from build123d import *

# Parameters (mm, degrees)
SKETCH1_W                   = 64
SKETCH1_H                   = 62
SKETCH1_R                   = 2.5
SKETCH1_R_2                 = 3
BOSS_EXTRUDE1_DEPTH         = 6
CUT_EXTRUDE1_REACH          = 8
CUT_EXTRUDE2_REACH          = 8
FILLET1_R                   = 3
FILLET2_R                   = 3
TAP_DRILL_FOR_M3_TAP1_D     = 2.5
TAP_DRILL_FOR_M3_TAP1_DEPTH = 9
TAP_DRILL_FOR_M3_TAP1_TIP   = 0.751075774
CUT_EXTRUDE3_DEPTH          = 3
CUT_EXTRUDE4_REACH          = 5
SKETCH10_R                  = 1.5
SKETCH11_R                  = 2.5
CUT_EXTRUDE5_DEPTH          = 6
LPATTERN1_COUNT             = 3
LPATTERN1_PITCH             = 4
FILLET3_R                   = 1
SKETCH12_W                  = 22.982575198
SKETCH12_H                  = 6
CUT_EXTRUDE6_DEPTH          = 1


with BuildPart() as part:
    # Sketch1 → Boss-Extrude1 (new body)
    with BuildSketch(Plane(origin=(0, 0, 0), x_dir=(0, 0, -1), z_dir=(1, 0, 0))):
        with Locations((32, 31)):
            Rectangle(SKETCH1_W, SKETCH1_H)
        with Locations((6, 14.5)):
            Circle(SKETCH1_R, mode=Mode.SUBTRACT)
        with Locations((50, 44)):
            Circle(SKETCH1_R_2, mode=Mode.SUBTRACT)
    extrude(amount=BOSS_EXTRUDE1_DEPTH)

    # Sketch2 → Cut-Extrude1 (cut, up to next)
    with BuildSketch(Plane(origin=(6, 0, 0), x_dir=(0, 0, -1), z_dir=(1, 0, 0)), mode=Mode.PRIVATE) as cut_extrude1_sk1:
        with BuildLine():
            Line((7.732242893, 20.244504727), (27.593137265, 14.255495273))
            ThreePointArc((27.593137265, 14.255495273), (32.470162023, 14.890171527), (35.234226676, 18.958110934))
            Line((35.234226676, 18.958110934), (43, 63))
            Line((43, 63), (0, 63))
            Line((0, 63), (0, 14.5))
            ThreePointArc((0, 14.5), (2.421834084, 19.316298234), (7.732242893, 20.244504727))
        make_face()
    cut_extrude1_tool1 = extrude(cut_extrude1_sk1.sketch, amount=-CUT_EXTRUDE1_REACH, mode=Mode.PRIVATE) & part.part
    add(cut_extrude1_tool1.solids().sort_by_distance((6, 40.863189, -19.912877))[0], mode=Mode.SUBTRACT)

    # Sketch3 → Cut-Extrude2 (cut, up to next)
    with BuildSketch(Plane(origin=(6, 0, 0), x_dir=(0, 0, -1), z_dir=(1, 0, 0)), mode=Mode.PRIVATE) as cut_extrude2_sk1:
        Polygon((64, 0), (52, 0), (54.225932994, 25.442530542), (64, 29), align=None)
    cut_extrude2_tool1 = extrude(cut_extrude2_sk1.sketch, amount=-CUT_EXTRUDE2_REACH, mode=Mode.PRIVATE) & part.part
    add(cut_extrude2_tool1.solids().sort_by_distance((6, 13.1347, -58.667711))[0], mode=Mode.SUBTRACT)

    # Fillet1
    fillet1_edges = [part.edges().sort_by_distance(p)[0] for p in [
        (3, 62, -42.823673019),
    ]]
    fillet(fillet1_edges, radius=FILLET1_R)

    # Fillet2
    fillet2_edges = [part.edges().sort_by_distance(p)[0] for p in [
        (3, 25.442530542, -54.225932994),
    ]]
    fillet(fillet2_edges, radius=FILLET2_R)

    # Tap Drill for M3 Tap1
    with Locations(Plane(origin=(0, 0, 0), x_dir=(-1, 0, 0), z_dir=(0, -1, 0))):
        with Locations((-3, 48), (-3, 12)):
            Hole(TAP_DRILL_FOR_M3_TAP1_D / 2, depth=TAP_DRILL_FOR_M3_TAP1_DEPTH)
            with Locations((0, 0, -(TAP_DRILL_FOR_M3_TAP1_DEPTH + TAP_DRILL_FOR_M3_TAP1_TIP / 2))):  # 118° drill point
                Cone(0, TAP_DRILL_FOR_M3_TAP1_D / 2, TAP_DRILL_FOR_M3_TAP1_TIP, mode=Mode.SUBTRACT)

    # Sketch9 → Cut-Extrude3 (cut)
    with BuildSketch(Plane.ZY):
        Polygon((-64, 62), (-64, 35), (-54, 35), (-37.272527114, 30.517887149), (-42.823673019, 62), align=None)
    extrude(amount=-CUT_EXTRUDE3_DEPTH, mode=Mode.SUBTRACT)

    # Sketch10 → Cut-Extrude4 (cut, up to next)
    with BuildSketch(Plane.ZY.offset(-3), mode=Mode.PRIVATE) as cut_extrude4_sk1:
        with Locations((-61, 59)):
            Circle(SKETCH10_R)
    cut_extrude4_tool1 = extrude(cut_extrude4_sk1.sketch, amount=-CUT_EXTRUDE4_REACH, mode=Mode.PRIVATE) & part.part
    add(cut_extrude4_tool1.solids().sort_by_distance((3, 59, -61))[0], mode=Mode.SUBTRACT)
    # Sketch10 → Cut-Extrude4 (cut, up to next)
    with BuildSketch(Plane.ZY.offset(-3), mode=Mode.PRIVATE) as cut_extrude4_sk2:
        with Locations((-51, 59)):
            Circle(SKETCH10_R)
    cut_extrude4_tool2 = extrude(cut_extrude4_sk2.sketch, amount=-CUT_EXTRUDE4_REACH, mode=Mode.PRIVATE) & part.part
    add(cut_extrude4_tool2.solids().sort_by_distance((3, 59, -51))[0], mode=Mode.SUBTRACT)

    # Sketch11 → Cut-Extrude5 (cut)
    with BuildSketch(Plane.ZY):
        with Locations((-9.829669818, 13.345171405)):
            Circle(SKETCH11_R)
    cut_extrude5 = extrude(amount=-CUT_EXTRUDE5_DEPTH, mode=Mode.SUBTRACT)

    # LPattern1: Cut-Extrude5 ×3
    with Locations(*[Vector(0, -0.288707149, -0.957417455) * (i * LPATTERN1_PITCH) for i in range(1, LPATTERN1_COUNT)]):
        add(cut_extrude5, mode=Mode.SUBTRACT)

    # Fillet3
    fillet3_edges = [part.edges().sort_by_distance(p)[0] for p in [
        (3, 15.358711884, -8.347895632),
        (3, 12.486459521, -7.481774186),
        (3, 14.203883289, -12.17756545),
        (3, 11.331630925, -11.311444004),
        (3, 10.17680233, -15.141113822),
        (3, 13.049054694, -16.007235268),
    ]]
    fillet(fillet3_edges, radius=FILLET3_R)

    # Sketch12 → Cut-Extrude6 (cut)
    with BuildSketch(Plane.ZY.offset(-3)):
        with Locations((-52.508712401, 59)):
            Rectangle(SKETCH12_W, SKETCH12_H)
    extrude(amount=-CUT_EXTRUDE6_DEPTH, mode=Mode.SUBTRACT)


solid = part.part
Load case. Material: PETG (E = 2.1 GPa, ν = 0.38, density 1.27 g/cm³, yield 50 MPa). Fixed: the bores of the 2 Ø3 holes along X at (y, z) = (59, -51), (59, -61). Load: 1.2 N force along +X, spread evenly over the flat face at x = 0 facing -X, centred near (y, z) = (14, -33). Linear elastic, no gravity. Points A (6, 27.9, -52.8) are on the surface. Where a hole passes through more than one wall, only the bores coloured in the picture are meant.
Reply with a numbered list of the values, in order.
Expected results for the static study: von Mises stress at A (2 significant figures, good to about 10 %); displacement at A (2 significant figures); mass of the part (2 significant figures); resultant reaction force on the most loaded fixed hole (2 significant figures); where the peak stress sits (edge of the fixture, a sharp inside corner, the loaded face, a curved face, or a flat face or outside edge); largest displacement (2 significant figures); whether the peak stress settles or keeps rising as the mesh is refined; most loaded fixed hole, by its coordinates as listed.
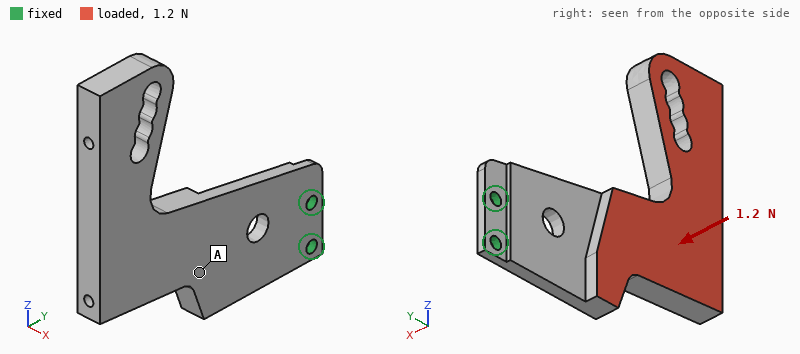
1. 0.37 MPa
2. 0.30 mm
3. 11 g
4. 3.0 N
5. edge of the fixture
6. 0.93 mm
7. keeps rising
8. (59, -51)
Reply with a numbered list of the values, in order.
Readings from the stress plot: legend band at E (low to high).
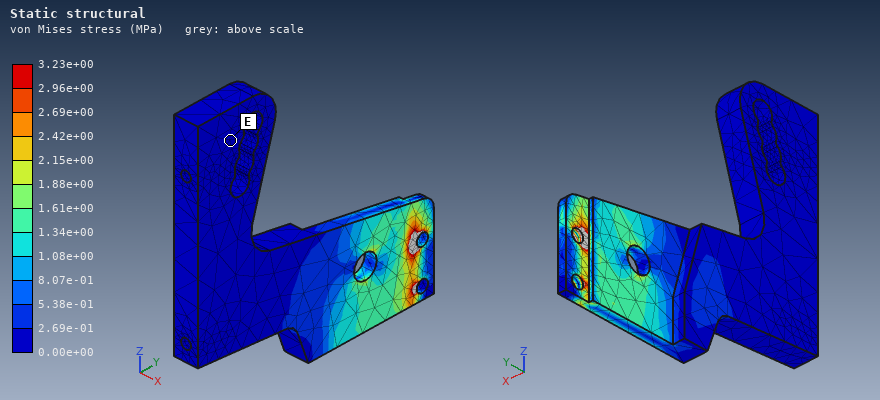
1. 0.00e+00 to 2.69e-01 MPa
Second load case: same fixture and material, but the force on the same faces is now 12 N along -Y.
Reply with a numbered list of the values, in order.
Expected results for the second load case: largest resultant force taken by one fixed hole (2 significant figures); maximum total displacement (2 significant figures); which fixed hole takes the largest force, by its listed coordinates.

1. 29 N
2. 1.0 mm
3. (59, -51)
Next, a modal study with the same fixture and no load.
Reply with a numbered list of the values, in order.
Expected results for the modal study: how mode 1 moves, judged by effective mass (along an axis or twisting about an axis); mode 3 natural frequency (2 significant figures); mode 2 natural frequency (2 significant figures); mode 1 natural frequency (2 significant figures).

1. along X
2. 410 Hz
3. 280 Hz
4. 73 Hz
